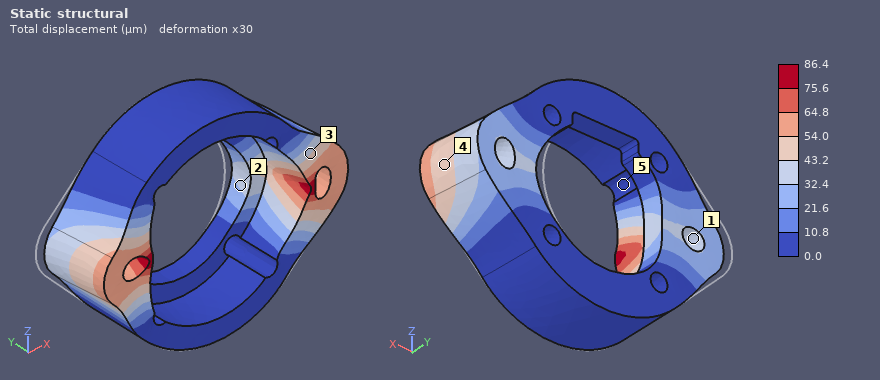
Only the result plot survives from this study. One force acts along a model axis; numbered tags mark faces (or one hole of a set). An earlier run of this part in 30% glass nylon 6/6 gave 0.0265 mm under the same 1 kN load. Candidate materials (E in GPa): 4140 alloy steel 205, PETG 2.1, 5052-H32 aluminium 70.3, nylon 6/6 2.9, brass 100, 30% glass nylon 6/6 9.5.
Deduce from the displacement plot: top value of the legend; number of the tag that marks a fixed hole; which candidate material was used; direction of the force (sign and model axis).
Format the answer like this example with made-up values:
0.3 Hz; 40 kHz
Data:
86.4 µm; 5; nylon 6/6; +X
